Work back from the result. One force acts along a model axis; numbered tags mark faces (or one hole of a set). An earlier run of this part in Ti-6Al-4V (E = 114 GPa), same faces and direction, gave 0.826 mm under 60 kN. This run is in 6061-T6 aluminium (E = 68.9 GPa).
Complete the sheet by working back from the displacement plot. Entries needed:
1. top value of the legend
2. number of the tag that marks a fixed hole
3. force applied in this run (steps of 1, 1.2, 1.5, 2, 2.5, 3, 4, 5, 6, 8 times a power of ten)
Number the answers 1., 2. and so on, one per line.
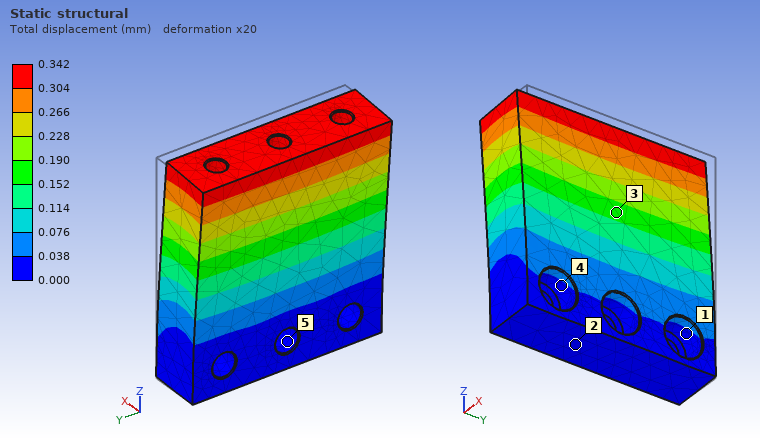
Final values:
1. 0.342 mm
2. 5
3. 15 kN
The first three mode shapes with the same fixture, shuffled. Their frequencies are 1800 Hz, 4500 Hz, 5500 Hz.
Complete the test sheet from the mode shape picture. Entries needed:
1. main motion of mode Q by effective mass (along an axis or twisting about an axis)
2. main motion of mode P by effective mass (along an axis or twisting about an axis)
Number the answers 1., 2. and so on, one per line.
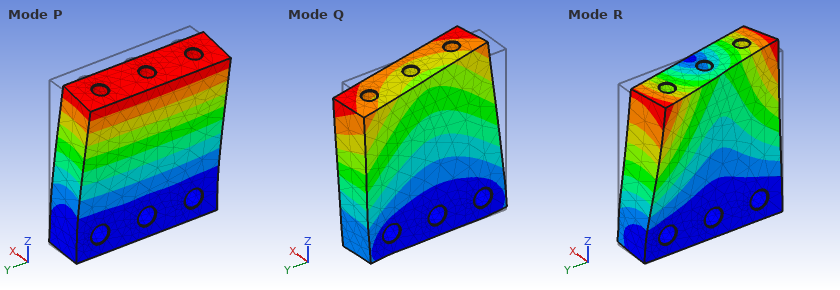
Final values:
1. along Y
2. along X
